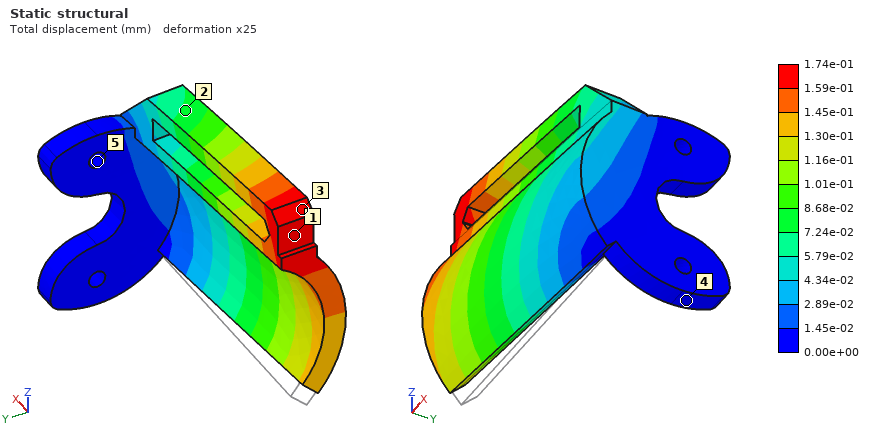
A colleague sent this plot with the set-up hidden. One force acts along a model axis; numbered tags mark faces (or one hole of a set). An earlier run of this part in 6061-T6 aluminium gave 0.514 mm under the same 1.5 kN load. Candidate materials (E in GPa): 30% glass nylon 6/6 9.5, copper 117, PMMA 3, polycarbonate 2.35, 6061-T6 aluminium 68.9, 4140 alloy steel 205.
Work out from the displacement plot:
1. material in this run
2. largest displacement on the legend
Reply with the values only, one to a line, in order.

4140 alloy steel
1.74e-01 mm
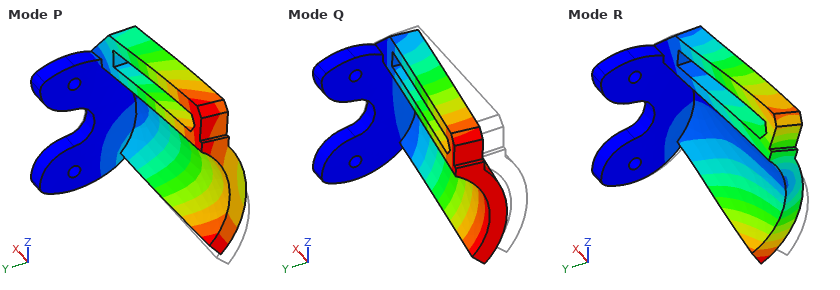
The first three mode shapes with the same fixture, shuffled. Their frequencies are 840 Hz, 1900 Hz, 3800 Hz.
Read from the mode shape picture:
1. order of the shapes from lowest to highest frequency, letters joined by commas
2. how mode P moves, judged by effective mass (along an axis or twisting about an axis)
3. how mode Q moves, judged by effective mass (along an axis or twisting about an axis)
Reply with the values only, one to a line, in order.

Q, P, R
along Z
along Y
